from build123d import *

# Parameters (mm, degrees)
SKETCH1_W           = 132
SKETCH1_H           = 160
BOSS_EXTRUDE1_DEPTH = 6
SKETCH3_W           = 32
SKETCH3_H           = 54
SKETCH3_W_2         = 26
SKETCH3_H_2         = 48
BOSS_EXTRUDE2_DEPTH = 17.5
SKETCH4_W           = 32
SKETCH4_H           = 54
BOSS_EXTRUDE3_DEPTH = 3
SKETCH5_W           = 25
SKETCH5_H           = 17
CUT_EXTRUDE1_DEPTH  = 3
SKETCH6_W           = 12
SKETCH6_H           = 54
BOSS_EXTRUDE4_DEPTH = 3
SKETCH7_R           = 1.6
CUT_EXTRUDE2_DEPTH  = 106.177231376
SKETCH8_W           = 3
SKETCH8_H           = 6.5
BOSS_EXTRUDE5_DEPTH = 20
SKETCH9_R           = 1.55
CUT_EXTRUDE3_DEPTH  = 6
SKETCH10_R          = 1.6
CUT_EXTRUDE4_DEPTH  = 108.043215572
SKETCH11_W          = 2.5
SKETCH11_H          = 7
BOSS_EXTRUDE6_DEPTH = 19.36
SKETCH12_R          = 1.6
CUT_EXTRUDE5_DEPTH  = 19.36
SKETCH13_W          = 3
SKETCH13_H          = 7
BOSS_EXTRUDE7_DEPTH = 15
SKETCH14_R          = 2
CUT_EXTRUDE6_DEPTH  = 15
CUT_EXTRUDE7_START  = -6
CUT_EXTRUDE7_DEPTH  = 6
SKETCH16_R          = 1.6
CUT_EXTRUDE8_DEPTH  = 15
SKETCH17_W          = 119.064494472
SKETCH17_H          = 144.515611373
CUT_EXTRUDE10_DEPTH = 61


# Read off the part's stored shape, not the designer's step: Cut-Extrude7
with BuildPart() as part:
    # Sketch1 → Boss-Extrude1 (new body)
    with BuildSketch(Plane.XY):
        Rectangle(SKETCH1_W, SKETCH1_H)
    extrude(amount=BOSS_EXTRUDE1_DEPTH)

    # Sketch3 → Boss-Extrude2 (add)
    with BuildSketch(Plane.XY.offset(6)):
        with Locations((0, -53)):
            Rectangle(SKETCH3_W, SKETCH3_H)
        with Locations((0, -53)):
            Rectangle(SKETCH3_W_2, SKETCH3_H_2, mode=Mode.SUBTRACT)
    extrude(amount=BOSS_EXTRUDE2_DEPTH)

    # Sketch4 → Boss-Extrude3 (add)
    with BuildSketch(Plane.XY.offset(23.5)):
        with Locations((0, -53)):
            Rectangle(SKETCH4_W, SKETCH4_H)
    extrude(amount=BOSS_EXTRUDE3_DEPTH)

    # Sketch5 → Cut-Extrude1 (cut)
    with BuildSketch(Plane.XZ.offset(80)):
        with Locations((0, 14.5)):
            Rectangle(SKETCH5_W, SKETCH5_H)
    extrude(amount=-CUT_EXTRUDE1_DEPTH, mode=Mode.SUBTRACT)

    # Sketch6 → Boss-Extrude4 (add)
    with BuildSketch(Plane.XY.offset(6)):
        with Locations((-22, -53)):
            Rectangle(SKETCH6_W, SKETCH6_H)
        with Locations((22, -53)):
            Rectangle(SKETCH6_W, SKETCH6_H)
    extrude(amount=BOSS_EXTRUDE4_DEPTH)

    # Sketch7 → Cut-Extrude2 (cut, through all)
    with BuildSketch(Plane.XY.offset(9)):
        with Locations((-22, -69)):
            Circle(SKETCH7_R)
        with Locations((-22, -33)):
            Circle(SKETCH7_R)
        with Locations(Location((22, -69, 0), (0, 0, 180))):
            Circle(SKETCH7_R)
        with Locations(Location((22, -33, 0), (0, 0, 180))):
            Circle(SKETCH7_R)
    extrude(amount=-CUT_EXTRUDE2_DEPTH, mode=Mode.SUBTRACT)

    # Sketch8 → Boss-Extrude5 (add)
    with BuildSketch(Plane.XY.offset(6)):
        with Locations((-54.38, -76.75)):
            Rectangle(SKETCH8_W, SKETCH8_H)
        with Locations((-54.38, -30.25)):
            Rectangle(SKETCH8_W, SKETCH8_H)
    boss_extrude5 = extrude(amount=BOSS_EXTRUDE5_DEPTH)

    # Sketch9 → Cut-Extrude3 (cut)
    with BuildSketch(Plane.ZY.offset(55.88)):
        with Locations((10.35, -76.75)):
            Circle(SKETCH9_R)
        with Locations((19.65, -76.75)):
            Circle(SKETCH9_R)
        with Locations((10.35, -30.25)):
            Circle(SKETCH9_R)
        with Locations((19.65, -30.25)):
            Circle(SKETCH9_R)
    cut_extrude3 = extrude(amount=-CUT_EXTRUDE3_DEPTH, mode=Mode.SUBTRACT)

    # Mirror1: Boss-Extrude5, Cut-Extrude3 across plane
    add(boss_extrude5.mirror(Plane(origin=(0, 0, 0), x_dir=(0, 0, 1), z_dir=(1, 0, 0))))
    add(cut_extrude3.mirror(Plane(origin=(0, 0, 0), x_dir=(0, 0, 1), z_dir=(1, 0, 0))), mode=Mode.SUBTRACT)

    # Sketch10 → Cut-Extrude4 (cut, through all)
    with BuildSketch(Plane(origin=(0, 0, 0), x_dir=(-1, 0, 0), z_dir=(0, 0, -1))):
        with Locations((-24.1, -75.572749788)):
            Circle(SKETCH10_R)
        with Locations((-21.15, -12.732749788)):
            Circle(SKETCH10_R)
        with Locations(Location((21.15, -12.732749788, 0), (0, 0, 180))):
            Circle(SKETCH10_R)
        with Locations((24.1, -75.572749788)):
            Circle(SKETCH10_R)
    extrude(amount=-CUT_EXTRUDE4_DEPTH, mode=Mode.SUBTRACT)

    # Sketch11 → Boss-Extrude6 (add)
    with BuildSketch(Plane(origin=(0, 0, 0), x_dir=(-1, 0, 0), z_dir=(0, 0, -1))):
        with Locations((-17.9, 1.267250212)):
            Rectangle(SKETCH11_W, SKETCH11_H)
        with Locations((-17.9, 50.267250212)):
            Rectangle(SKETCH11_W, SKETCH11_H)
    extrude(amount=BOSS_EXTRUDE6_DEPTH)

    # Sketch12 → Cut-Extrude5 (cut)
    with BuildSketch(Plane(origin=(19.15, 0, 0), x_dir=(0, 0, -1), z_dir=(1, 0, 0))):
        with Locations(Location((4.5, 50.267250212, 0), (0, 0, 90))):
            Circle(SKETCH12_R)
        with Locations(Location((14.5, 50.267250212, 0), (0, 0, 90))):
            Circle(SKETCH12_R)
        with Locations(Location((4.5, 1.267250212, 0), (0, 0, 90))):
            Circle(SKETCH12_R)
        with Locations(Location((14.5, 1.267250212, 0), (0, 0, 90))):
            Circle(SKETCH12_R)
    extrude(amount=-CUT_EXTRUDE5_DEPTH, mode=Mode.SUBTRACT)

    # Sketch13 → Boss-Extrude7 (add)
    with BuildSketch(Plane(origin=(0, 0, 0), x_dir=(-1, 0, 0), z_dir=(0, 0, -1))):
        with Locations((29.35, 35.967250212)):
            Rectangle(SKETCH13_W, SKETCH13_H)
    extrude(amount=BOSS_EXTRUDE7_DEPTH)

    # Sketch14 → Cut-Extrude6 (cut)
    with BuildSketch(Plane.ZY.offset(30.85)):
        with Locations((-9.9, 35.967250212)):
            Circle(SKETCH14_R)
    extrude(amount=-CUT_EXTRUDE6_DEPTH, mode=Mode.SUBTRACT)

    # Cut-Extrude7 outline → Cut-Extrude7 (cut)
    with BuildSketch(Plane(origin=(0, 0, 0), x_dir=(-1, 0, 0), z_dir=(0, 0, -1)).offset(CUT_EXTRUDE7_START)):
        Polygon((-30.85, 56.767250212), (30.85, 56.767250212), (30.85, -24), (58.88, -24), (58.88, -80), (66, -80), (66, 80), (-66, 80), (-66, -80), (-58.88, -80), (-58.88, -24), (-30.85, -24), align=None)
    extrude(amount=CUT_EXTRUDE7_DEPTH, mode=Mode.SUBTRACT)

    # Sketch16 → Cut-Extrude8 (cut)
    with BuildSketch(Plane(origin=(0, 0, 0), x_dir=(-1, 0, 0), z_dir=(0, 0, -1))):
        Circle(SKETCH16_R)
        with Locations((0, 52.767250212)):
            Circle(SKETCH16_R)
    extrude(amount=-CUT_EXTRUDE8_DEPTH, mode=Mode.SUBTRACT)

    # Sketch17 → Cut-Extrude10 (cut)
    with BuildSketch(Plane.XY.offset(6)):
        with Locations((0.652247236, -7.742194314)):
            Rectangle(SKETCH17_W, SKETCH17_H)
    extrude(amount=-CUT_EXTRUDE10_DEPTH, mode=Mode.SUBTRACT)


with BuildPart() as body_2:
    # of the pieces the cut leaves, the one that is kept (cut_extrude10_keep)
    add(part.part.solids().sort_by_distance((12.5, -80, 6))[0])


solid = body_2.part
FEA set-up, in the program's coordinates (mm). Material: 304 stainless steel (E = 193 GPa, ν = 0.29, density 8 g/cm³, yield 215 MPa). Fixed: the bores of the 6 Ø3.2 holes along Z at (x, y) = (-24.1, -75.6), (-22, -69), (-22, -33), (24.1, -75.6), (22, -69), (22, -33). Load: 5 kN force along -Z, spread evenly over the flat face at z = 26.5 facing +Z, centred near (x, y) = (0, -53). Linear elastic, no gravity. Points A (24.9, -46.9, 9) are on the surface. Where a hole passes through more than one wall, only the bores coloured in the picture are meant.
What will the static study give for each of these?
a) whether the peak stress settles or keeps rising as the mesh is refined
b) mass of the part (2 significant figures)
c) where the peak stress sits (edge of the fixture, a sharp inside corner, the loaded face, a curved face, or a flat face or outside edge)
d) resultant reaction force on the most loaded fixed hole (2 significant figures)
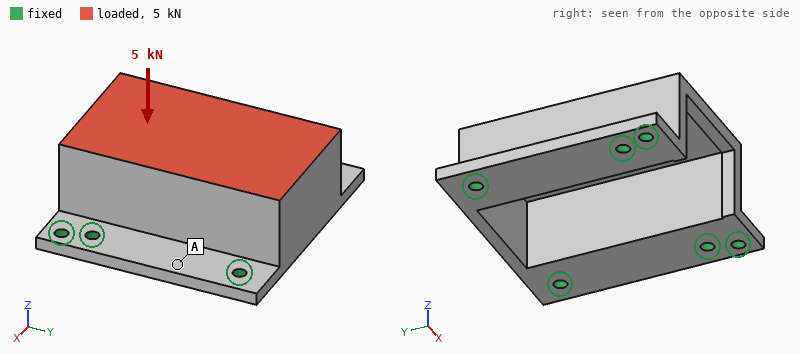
keeps rising
130 g
edge of the fixture
1.3 kN
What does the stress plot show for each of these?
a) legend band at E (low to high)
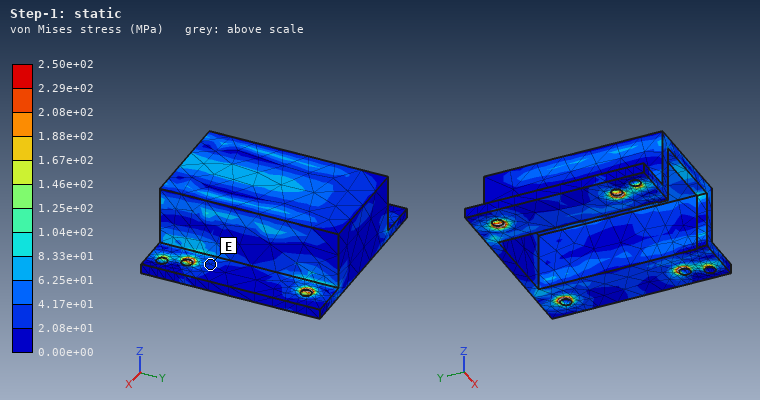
2.08e+01 to 4.17e+01 MPa
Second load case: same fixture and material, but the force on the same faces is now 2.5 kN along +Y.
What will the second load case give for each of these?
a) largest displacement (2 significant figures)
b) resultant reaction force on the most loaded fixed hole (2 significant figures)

14 µm
890 N
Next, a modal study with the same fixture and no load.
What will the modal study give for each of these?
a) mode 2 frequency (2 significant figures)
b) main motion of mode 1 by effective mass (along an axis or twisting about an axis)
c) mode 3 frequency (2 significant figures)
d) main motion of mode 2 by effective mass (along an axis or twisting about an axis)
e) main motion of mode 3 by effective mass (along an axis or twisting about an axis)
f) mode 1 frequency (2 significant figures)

8300 Hz
along X
9500 Hz
along Y
along Z
5500 Hz
